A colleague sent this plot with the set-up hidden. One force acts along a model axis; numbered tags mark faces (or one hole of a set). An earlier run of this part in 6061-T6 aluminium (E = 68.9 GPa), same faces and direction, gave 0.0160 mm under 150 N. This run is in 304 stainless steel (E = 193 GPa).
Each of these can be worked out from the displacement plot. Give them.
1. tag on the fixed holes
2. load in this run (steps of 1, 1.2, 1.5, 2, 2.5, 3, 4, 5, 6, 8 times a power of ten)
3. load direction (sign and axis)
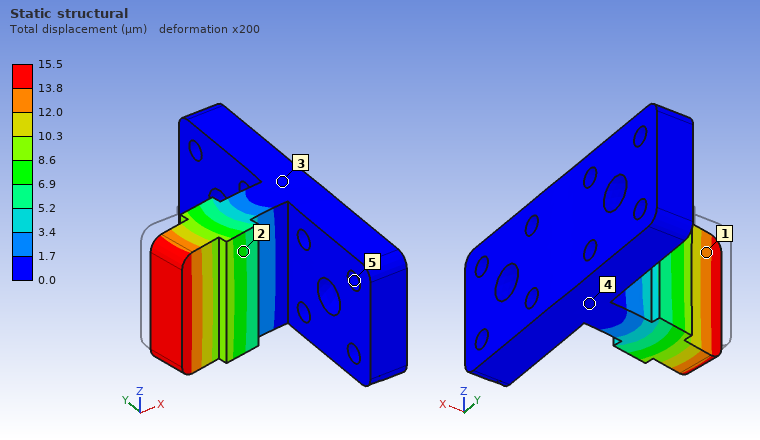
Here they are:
5
400 N
-Y
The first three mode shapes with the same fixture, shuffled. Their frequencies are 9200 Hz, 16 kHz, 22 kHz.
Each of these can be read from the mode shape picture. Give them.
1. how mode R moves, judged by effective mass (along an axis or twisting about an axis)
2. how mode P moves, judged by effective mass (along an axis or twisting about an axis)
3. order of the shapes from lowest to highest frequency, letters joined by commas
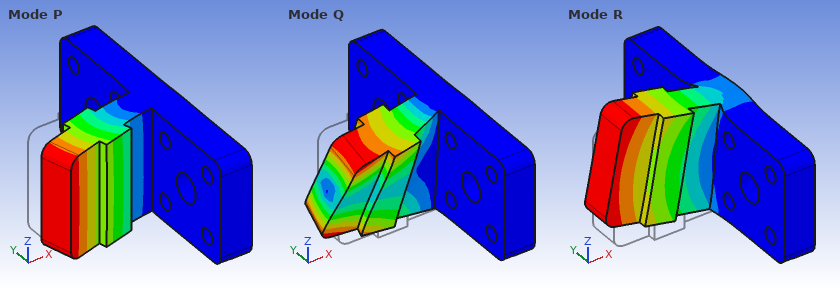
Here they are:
along Z
along Y
P, R, Q
